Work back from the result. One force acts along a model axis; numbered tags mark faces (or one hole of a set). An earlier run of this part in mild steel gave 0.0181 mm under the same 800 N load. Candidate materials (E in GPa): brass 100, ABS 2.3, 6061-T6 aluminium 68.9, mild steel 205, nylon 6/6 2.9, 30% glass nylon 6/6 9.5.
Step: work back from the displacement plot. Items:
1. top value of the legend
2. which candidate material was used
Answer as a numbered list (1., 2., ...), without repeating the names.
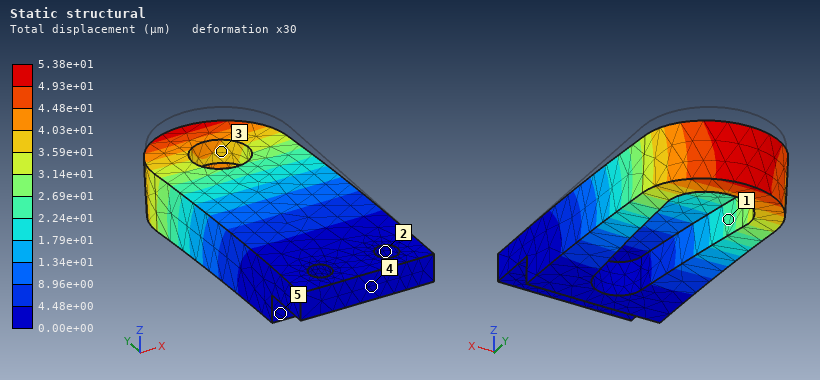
1. 5.38e+01 µm
2. 6061-T6 aluminium
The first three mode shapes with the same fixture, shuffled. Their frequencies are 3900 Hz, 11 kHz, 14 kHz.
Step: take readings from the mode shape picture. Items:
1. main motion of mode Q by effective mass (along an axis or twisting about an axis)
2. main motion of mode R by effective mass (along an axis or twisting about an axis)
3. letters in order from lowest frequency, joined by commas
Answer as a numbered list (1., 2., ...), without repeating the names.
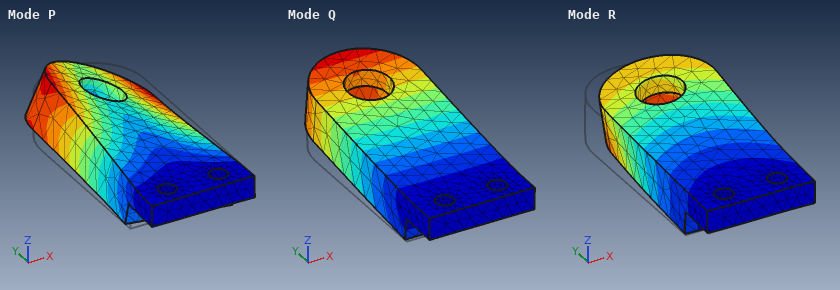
1. along Z
2. along X
3. Q, R, P
